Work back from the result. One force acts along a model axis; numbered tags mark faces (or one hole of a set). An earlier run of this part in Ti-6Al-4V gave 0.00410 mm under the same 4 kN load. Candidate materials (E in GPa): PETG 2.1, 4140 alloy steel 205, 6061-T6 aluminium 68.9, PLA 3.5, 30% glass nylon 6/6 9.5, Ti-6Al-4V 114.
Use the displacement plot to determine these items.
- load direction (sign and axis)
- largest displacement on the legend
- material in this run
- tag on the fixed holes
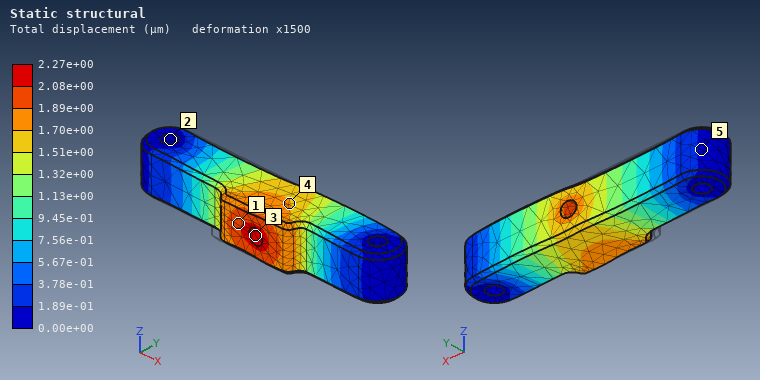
+X
2.27e+00 µm
4140 alloy steel
2
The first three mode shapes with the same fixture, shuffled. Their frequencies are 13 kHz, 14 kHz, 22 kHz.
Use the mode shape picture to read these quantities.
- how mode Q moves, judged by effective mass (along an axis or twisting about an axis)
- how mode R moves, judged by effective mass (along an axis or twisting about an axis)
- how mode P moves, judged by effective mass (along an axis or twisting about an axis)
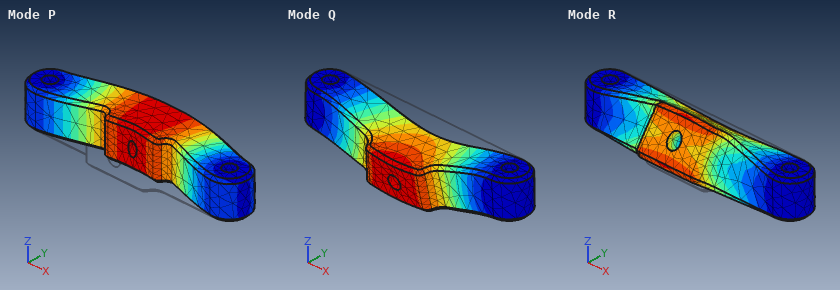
along Z
twisting about X
along Y
